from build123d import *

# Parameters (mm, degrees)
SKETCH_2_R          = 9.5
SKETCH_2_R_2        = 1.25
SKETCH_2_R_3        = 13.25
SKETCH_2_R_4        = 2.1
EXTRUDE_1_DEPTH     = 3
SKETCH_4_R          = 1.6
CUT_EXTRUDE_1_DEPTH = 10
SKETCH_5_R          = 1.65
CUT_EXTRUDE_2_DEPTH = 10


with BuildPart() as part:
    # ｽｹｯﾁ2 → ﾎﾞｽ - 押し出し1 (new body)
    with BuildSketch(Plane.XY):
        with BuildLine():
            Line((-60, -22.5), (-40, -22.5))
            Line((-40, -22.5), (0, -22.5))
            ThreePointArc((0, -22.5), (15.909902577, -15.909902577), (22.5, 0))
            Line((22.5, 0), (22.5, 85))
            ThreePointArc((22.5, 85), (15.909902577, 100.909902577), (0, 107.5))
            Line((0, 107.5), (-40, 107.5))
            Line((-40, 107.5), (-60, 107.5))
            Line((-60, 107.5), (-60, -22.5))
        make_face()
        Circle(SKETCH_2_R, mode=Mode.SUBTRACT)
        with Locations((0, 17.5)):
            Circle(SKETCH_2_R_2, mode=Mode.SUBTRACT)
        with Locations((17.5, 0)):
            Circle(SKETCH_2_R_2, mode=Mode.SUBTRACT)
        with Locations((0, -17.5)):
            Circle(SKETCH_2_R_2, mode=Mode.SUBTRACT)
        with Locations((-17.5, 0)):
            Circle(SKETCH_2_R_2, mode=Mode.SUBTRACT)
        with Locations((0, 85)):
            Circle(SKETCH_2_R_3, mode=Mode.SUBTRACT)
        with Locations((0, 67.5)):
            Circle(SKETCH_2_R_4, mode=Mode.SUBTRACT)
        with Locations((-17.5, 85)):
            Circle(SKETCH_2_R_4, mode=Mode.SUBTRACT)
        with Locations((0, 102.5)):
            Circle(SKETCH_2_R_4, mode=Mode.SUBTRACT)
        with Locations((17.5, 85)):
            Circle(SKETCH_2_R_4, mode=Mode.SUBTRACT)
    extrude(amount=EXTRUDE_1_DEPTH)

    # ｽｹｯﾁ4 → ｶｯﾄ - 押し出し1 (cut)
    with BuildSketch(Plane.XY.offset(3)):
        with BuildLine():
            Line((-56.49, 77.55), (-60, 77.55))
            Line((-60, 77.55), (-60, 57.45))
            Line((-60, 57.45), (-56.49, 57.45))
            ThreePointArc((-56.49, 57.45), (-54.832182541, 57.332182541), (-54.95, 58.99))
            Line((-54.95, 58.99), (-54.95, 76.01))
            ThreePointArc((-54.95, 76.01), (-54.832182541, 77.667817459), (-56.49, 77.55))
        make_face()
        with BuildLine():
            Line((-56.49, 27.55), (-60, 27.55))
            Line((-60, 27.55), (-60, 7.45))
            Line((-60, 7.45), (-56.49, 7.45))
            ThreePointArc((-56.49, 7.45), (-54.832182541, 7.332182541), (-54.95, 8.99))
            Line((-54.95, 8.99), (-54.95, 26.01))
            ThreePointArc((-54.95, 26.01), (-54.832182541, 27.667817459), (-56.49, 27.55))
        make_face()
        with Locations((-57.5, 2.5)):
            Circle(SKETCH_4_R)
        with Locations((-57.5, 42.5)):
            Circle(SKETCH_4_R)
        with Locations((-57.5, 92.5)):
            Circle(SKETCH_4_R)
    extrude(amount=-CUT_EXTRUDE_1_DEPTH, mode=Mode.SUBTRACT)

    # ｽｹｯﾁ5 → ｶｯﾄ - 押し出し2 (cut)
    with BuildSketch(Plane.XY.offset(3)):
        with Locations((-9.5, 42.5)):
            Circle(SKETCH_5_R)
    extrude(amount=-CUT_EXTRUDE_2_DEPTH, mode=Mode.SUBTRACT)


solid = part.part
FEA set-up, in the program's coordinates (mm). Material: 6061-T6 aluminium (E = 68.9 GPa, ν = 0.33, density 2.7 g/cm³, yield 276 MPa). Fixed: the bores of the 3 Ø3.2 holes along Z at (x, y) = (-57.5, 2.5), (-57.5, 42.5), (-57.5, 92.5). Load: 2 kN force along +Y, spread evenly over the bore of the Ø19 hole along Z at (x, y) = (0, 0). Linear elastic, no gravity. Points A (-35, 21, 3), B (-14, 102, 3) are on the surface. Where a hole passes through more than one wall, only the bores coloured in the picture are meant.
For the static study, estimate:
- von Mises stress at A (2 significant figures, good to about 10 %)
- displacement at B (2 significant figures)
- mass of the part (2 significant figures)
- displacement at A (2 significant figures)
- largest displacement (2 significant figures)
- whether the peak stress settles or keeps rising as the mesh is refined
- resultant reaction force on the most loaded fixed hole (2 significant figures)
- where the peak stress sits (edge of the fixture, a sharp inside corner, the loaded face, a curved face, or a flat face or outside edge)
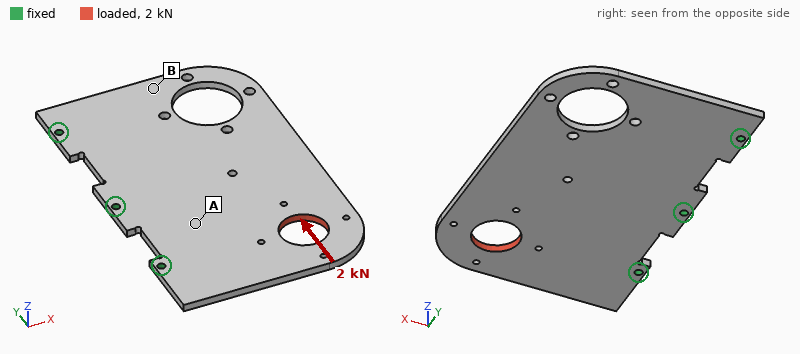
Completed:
18 MPa
21 µm
76 g
14 µm
49 µm
keeps rising
1.4 kN
edge of the fixture
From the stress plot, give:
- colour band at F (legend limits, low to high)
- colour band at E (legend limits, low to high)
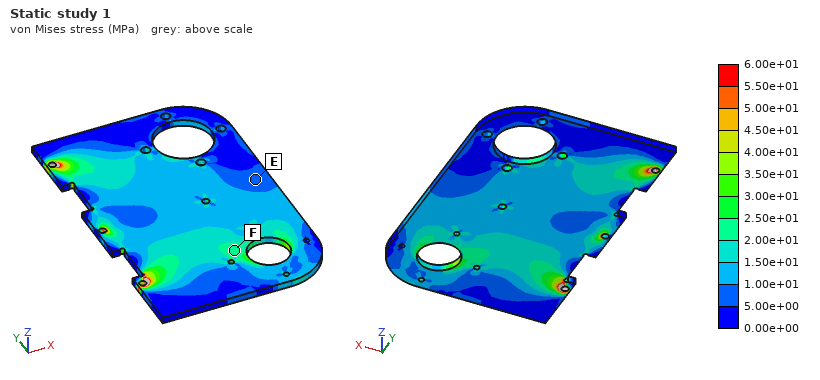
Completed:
2.00e+01 to 2.50e+01 MPa
5.00e+00 to 1.00e+01 MPa
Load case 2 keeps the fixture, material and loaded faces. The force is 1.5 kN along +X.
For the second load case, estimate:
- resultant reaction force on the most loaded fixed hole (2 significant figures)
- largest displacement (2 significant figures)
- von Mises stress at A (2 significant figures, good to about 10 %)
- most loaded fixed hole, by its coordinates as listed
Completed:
1.3 kN
24 µm
5.8 MPa
(-57.5, 2.5)
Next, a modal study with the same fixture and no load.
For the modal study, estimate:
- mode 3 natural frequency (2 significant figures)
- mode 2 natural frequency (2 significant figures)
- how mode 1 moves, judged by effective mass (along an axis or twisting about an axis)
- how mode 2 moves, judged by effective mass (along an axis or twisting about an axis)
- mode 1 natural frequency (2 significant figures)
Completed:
1400 Hz
700 Hz
along Z
twisting about X
350 Hz
